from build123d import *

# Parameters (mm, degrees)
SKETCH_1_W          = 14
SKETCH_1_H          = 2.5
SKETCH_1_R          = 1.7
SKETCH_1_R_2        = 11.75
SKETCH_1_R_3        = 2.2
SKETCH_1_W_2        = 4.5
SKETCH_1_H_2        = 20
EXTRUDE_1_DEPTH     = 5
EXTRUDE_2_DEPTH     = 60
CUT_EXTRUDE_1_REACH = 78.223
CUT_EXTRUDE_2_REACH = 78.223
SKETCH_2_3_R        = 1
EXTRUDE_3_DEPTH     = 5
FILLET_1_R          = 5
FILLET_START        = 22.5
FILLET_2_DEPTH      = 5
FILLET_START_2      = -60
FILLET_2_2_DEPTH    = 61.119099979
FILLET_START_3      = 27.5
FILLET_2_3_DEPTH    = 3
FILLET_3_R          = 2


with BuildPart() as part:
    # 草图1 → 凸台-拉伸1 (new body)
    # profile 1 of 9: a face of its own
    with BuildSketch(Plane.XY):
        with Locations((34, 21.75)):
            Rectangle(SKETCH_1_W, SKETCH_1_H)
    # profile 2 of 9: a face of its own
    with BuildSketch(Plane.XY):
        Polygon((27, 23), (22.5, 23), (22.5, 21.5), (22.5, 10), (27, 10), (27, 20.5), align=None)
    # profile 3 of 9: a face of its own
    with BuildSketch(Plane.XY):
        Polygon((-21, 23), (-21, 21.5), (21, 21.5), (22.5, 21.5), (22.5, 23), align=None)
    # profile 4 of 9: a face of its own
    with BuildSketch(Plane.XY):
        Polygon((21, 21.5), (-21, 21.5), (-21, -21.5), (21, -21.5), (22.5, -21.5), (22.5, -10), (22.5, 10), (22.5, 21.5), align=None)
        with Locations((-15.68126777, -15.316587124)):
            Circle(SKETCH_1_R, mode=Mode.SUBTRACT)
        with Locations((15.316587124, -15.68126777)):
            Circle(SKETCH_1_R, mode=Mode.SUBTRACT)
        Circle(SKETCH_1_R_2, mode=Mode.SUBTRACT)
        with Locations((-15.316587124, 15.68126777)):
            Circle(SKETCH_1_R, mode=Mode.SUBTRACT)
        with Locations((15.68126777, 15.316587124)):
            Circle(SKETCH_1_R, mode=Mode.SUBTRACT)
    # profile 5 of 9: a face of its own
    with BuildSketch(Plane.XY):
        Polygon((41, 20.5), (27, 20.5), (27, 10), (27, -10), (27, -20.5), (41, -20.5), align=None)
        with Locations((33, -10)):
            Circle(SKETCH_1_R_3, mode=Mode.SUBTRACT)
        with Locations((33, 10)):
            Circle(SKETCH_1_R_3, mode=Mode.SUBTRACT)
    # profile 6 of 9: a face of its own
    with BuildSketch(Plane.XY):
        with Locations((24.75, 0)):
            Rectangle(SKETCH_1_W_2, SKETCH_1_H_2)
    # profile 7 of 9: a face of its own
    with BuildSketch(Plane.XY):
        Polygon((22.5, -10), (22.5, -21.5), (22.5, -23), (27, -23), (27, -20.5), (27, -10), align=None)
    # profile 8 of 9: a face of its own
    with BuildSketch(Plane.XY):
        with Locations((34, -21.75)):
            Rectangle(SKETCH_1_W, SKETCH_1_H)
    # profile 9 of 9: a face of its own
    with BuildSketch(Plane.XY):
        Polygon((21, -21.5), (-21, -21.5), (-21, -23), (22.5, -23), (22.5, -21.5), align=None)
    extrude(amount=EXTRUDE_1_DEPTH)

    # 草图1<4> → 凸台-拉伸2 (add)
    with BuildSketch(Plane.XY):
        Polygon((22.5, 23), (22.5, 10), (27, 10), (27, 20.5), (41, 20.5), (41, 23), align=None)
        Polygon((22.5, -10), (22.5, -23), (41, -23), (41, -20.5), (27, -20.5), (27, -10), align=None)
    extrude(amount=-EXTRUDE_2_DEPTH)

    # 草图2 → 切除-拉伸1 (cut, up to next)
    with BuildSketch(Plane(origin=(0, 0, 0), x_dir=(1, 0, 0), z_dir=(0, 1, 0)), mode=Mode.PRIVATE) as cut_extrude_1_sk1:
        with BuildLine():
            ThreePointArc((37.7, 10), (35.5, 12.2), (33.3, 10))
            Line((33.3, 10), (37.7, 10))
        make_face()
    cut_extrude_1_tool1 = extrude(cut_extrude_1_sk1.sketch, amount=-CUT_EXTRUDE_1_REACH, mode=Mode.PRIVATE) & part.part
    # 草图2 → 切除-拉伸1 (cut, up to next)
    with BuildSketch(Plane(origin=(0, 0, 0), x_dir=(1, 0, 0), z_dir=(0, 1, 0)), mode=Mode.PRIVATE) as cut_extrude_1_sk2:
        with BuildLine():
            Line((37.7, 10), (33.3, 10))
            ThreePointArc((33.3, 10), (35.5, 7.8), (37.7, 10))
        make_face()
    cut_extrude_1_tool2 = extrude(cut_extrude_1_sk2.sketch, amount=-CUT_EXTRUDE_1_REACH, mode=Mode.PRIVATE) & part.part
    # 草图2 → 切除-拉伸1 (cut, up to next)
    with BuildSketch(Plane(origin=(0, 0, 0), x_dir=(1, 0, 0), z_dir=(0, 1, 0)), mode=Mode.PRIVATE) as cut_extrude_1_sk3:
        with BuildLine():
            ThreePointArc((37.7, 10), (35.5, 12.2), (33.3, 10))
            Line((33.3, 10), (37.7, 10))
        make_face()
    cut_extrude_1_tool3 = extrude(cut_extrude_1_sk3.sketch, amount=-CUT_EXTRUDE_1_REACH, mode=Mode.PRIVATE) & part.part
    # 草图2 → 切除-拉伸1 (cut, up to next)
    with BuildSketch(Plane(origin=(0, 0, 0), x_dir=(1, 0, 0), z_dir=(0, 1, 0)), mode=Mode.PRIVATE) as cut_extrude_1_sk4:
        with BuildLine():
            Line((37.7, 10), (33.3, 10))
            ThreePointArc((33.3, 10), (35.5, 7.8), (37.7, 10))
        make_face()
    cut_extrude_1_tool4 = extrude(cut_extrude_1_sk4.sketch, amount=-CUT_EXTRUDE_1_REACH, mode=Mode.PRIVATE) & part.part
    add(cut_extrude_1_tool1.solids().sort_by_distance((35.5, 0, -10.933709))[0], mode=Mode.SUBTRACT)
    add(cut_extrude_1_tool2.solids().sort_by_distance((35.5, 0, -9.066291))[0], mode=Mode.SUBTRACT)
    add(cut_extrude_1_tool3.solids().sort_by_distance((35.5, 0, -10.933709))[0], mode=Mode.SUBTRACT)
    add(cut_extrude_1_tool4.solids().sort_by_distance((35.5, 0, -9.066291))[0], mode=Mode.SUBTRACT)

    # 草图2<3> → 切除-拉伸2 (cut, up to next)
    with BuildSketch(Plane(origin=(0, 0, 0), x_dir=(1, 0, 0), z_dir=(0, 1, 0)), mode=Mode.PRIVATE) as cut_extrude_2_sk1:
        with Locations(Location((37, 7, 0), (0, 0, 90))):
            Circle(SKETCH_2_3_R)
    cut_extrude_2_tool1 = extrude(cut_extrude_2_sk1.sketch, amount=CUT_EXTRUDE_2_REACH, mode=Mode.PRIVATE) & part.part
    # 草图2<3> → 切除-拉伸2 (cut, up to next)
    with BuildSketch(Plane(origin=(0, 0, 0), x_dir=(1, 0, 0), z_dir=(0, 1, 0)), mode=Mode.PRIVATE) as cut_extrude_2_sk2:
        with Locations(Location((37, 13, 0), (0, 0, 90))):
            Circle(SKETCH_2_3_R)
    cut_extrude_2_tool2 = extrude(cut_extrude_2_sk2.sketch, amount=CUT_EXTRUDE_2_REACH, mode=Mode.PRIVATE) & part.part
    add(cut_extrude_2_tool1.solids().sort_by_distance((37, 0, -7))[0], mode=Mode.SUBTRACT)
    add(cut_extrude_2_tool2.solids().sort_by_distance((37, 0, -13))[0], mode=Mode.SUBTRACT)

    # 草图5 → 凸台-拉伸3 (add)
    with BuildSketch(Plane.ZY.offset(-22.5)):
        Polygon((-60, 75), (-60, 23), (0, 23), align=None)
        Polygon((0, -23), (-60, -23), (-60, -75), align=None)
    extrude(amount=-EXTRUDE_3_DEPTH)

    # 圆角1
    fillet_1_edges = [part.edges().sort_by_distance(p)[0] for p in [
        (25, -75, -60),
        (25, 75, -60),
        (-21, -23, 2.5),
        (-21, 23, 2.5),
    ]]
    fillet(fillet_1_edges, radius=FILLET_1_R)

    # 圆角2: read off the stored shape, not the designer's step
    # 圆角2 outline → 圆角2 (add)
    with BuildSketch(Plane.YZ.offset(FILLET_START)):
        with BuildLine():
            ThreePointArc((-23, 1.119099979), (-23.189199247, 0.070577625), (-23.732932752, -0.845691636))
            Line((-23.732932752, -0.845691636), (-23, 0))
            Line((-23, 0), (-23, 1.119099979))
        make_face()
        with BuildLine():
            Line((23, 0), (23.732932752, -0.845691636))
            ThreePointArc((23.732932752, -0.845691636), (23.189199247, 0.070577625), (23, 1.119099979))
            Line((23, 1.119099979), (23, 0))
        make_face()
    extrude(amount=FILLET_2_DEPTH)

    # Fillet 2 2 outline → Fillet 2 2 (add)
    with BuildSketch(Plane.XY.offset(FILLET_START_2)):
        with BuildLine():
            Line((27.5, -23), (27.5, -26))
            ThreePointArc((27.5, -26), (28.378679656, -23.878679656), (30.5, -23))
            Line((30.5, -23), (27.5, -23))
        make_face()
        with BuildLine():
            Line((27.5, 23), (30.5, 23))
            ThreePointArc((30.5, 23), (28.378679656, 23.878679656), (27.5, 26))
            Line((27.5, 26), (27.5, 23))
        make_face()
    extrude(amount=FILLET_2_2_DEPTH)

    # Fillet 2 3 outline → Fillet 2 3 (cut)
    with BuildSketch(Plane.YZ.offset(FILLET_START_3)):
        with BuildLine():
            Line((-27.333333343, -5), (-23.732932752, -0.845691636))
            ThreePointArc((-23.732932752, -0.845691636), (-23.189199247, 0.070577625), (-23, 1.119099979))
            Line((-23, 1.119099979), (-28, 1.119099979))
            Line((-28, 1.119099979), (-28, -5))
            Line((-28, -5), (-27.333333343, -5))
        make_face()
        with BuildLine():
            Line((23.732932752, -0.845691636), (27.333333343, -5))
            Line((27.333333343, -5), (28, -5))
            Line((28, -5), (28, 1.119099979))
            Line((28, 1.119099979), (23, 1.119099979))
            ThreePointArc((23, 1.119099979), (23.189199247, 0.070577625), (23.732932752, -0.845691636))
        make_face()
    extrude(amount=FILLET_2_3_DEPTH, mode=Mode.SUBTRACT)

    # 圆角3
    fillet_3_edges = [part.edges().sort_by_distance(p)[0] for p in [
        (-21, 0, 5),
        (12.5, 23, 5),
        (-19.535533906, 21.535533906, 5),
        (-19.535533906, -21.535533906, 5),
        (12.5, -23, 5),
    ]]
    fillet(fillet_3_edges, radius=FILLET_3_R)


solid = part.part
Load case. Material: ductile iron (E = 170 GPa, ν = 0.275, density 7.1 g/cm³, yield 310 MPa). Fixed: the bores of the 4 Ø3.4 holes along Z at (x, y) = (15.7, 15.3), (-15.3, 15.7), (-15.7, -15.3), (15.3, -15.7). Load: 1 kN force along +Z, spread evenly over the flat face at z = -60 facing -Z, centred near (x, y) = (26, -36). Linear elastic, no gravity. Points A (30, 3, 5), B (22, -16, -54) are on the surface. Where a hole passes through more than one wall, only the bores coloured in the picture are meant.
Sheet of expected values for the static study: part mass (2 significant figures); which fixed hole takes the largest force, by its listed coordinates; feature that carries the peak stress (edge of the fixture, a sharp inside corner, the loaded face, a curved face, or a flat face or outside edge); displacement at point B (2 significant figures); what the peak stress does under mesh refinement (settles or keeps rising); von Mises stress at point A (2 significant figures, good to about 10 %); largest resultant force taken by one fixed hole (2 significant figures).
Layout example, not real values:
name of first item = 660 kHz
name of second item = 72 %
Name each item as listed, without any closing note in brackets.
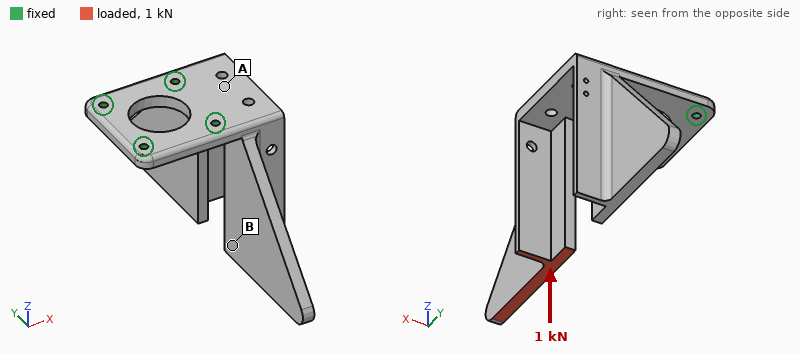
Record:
part mass = 270 g
which fixed hole takes the largest force, by its listed coordinates = (15.3, -15.7)
feature that carries the peak stress = edge of the fixture
displacement at point B = 0.21 mm
what the peak stress does under mesh refinement = keeps rising
von Mises stress at point A = 40 MPa
largest resultant force taken by one fixed hole = 1.4 kN
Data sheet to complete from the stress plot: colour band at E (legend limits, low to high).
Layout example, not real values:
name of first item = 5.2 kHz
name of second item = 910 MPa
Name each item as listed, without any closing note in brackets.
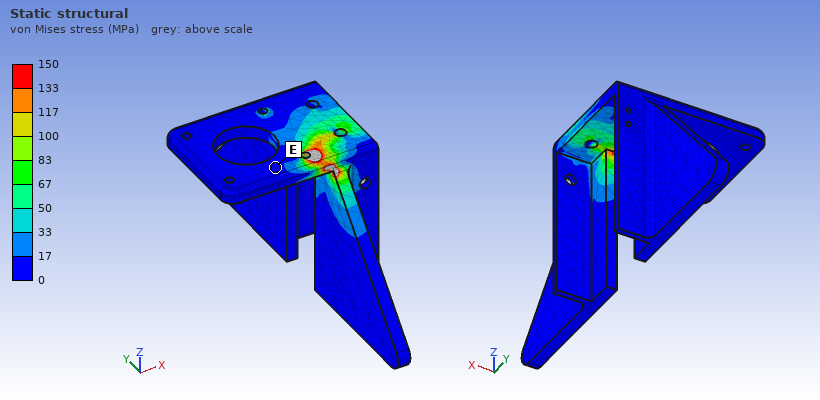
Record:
colour band at E = 0 to 17 MPa
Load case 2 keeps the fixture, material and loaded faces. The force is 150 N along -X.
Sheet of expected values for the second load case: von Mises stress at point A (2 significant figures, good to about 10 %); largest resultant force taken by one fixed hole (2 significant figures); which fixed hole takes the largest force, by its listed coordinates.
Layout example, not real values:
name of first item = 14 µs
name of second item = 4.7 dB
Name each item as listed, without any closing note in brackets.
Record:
von Mises stress at point A = 30 MPa
largest resultant force taken by one fixed hole = 220 N
which fixed hole takes the largest force, by its listed coordinates = (15.3, -15.7)
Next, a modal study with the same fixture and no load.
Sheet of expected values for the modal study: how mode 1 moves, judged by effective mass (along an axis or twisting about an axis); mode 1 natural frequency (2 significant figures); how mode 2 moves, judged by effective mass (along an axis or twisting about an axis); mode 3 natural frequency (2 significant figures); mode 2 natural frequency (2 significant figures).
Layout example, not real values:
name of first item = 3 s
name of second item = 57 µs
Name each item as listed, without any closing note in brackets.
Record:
how mode 1 moves, judged by effective mass = along X
mode 1 natural frequency = 570 Hz
how mode 2 moves, judged by effective mass = twisting about Z
mode 3 natural frequency = 840 Hz
mode 2 natural frequency = 670 Hz
